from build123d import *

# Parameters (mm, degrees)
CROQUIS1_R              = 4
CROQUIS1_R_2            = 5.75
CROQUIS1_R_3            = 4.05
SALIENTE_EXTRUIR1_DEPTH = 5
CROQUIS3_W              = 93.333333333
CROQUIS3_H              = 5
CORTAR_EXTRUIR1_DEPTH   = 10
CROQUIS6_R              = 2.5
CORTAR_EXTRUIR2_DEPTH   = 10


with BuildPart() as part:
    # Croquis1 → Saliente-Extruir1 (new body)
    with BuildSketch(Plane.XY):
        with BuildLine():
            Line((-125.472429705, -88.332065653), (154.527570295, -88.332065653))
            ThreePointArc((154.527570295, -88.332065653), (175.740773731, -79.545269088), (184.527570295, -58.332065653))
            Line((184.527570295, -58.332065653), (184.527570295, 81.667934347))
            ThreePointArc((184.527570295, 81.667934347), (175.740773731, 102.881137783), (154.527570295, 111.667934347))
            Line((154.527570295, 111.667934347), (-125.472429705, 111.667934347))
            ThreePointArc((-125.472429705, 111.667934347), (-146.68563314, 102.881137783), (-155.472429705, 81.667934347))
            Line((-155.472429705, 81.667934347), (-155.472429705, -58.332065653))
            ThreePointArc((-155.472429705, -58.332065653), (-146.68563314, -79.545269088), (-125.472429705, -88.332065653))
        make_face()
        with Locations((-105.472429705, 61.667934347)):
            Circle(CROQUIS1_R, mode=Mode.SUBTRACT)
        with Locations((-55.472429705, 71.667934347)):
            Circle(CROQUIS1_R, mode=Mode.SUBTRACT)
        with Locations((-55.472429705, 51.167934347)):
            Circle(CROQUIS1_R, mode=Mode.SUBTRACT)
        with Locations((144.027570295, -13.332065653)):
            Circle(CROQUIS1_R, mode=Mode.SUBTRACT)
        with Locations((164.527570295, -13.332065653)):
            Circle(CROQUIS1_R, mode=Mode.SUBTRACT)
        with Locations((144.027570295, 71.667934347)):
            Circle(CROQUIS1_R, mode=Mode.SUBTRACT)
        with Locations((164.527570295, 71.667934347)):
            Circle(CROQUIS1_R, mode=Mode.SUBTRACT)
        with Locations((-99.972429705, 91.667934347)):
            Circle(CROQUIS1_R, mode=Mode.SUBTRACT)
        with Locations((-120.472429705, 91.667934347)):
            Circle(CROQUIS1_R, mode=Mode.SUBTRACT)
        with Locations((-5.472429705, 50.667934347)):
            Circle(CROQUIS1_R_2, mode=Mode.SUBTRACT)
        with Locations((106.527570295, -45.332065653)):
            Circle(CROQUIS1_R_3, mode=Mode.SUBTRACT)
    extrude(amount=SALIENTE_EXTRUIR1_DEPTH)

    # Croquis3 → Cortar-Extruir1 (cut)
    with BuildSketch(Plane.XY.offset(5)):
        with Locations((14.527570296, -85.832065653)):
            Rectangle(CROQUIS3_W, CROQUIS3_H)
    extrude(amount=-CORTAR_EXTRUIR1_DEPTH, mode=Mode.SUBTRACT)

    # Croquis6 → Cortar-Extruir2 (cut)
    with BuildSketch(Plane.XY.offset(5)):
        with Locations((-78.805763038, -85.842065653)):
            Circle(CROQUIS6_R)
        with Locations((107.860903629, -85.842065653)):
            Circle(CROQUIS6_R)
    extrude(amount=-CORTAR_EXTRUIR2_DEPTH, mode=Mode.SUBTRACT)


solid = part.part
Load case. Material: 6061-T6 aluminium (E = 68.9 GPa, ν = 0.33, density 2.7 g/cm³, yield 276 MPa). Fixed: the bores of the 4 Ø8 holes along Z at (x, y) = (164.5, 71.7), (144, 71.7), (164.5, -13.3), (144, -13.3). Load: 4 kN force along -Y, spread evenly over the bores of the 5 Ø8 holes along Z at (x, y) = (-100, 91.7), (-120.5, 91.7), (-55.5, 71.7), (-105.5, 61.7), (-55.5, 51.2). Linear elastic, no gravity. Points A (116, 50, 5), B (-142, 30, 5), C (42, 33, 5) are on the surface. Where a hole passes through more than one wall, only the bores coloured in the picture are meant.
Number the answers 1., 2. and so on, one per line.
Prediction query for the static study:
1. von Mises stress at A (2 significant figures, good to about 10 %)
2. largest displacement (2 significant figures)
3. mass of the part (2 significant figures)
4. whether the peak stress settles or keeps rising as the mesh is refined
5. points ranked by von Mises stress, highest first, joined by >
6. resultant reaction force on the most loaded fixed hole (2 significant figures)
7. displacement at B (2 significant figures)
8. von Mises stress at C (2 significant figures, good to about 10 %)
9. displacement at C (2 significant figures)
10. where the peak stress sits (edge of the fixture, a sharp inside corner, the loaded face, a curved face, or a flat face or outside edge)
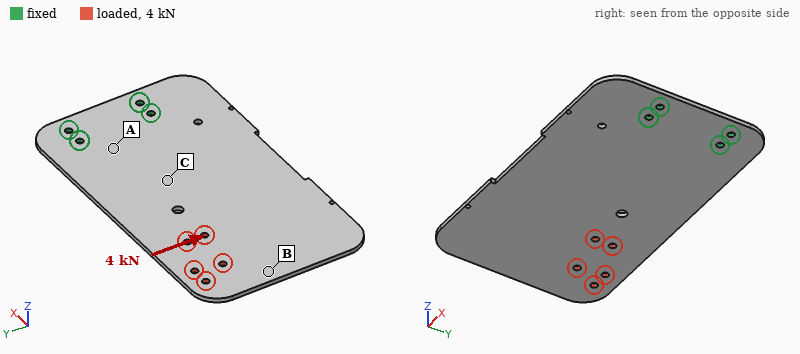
1. 25 MPa
2. 0.30 mm
3. 890 g
4. keeps rising
5. A > C > B
6. 7.5 kN
7. 0.27 mm
8. 13 MPa
9. 0.085 mm
10. edge of the fixture
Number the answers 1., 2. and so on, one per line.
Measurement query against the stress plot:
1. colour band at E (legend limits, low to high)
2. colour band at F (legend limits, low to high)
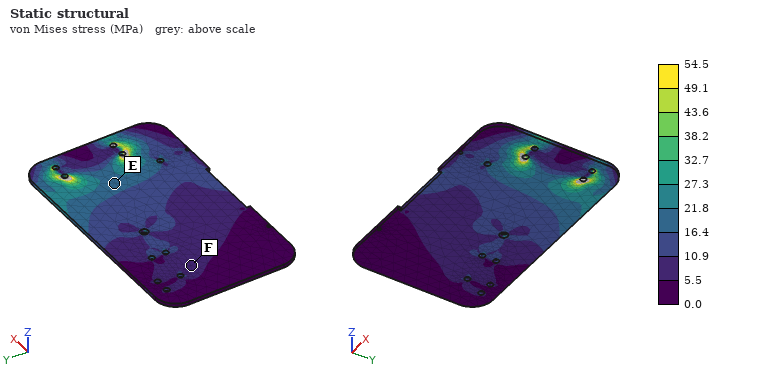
1. 16.4 to 21.8 MPa
2. 5.5 to 10.9 MPa
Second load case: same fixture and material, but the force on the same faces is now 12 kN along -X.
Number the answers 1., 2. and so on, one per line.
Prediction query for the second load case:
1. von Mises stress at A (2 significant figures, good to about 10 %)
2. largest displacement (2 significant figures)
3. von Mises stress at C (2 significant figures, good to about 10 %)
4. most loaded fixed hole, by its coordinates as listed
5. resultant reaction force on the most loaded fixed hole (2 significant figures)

1. 24 MPa
2. 0.23 mm
3. 17 MPa
4. (144, 71.7)
5. 8.0 kN
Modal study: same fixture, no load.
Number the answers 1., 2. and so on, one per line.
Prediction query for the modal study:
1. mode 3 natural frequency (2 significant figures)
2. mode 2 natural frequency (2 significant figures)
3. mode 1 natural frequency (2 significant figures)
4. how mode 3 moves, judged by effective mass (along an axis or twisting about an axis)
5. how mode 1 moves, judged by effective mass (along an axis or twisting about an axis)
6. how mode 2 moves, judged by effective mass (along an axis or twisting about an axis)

1. 280 Hz
2. 150 Hz
3. 45 Hz
4. along Z
5. along Z
6. twisting about X
